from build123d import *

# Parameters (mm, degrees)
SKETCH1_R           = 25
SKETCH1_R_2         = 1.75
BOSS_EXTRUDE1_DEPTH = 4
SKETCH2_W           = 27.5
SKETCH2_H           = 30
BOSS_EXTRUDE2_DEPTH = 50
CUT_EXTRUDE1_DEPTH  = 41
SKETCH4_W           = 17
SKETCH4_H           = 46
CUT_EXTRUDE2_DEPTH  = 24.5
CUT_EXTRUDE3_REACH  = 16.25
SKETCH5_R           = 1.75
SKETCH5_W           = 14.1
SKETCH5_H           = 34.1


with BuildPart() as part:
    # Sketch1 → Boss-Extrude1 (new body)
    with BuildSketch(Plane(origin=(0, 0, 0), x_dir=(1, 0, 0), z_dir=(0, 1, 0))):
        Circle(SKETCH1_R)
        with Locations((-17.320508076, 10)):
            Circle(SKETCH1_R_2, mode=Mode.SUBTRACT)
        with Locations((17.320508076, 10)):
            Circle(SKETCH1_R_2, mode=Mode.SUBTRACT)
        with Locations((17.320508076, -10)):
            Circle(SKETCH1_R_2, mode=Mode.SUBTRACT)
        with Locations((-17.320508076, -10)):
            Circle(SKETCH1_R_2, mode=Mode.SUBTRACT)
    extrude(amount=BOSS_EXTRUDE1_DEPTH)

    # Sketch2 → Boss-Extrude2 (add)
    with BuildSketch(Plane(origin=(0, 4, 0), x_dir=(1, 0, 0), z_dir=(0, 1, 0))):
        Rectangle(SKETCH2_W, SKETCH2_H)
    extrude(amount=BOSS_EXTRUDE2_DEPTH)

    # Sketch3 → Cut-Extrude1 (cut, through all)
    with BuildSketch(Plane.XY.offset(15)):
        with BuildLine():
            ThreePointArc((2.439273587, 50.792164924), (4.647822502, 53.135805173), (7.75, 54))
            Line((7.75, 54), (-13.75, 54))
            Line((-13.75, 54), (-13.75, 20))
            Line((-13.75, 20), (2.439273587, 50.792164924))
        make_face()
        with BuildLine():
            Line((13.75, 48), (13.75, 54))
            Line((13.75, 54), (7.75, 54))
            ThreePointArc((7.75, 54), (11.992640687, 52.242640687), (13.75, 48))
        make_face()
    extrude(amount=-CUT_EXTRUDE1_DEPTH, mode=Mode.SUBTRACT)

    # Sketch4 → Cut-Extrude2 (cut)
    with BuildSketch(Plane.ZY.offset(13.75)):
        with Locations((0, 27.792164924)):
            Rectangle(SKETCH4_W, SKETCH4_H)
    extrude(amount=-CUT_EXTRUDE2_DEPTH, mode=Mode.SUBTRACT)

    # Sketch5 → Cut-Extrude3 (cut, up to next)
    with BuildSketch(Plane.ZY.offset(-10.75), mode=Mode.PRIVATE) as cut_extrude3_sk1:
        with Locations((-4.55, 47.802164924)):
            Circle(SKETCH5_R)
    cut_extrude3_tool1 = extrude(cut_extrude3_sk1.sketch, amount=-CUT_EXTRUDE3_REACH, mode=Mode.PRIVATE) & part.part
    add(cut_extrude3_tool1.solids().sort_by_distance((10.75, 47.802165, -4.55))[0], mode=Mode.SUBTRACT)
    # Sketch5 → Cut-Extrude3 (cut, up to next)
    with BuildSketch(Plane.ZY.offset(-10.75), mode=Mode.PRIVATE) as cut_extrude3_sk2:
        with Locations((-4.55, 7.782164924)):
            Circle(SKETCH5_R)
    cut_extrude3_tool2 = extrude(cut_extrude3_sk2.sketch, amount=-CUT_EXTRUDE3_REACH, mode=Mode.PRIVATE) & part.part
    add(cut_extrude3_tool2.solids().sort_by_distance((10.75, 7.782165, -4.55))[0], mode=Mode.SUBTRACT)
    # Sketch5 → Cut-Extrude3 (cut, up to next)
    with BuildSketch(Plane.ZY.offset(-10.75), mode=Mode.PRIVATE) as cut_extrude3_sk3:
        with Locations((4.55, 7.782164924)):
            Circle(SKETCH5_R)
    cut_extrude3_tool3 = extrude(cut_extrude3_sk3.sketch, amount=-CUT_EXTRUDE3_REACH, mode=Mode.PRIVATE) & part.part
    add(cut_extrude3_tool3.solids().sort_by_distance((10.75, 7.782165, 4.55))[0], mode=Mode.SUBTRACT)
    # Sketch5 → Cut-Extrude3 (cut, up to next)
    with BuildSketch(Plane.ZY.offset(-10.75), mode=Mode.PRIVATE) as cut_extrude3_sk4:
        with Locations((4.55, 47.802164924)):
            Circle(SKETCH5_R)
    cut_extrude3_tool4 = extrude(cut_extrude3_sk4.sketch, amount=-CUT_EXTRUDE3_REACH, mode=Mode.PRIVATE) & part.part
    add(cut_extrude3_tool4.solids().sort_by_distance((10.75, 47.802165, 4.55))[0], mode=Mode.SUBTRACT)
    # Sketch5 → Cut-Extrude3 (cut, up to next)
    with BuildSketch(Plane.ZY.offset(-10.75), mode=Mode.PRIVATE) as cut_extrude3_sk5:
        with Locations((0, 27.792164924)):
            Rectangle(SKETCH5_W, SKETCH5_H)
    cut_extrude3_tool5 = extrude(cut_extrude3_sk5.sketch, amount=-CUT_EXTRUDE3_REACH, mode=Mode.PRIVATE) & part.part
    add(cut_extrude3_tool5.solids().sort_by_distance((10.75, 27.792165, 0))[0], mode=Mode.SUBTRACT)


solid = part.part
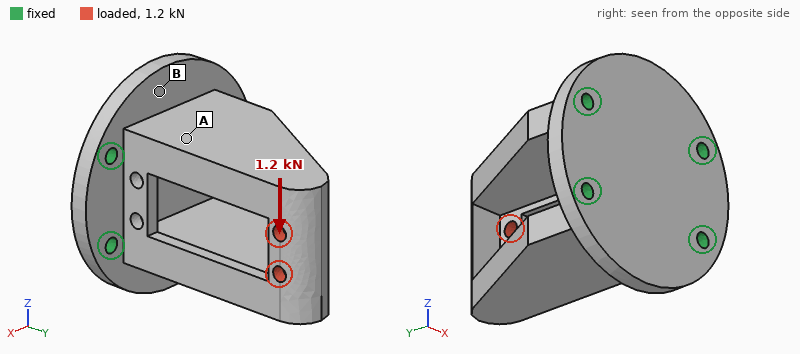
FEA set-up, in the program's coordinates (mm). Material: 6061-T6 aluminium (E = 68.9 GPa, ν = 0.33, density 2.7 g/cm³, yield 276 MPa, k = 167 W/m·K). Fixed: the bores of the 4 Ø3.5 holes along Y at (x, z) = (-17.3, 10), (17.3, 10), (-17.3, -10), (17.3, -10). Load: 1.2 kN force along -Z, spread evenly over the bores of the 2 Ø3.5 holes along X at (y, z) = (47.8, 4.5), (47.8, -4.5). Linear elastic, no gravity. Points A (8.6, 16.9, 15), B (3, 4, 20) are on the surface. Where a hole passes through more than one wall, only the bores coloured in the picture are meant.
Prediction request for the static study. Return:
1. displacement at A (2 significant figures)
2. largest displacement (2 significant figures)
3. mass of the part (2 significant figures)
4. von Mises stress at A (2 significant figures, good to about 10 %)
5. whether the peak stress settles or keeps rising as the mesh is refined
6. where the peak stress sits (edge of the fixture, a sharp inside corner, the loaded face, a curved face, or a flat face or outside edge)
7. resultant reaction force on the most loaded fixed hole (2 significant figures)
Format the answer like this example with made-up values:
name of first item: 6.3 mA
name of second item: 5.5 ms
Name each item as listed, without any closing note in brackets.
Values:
displacement at A: 0.073 mm
largest displacement: 0.34 mm
mass of the part: 62 g
von Mises stress at A: 65 MPa
whether the peak stress settles or keeps rising as the mesh is refined: keeps rising
where the peak stress sits: a sharp inside corner
resultant reaction force on the most loaded fixed hole: 1.4 kN
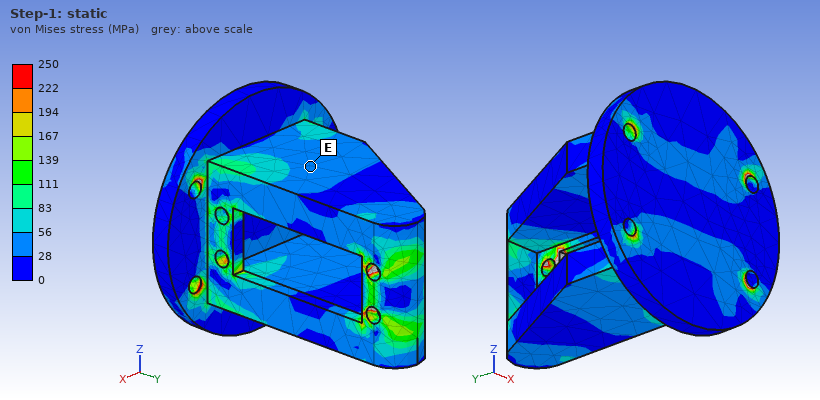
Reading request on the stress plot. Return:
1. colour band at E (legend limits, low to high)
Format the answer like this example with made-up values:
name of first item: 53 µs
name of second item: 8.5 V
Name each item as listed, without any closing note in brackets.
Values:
colour band at E: 28 to 56 MPa
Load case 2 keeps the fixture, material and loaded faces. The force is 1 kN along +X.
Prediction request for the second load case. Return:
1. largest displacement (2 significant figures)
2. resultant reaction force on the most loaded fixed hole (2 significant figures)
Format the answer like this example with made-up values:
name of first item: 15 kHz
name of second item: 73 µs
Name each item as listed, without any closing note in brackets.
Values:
largest displacement: 71 µm
resultant reaction force on the most loaded fixed hole: 810 N
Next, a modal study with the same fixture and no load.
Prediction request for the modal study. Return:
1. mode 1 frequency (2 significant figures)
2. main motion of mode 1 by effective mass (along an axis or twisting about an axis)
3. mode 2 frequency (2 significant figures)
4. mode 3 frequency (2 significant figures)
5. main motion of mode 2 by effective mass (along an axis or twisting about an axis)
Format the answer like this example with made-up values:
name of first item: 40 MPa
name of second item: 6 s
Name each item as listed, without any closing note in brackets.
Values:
mode 1 frequency: 2800 Hz
main motion of mode 1 by effective mass: along Z
mode 2 frequency: 6600 Hz
mode 3 frequency: 8000 Hz
main motion of mode 2 by effective mass: along X
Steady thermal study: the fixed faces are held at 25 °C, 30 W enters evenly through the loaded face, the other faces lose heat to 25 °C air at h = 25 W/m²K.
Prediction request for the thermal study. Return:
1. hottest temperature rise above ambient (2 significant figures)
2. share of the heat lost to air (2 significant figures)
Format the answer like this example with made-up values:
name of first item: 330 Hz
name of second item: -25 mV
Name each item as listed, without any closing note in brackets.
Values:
hottest temperature rise above ambient: 56 K
share of the heat lost to air: 11 %
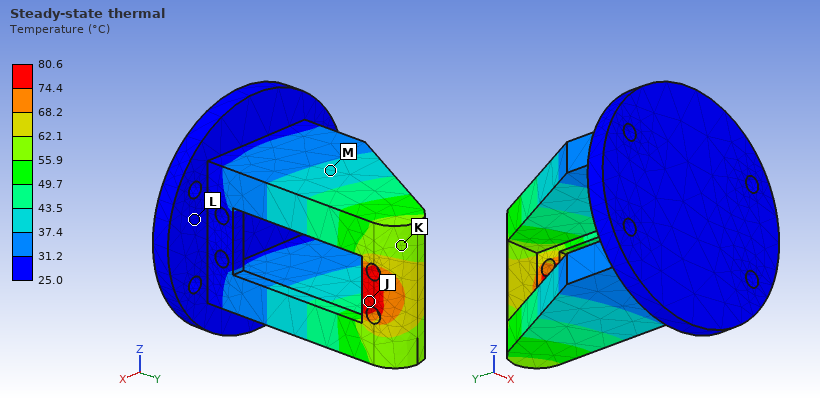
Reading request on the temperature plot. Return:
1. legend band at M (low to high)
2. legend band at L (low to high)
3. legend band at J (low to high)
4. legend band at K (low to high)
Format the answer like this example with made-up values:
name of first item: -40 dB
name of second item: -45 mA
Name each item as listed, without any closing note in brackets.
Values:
legend band at M: 37.4 to 43.5 °C
legend band at L: 25.0 to 31.2 °C
legend band at J: 74.4 to 80.6 °C
legend band at K: 55.9 to 62.1 °C
